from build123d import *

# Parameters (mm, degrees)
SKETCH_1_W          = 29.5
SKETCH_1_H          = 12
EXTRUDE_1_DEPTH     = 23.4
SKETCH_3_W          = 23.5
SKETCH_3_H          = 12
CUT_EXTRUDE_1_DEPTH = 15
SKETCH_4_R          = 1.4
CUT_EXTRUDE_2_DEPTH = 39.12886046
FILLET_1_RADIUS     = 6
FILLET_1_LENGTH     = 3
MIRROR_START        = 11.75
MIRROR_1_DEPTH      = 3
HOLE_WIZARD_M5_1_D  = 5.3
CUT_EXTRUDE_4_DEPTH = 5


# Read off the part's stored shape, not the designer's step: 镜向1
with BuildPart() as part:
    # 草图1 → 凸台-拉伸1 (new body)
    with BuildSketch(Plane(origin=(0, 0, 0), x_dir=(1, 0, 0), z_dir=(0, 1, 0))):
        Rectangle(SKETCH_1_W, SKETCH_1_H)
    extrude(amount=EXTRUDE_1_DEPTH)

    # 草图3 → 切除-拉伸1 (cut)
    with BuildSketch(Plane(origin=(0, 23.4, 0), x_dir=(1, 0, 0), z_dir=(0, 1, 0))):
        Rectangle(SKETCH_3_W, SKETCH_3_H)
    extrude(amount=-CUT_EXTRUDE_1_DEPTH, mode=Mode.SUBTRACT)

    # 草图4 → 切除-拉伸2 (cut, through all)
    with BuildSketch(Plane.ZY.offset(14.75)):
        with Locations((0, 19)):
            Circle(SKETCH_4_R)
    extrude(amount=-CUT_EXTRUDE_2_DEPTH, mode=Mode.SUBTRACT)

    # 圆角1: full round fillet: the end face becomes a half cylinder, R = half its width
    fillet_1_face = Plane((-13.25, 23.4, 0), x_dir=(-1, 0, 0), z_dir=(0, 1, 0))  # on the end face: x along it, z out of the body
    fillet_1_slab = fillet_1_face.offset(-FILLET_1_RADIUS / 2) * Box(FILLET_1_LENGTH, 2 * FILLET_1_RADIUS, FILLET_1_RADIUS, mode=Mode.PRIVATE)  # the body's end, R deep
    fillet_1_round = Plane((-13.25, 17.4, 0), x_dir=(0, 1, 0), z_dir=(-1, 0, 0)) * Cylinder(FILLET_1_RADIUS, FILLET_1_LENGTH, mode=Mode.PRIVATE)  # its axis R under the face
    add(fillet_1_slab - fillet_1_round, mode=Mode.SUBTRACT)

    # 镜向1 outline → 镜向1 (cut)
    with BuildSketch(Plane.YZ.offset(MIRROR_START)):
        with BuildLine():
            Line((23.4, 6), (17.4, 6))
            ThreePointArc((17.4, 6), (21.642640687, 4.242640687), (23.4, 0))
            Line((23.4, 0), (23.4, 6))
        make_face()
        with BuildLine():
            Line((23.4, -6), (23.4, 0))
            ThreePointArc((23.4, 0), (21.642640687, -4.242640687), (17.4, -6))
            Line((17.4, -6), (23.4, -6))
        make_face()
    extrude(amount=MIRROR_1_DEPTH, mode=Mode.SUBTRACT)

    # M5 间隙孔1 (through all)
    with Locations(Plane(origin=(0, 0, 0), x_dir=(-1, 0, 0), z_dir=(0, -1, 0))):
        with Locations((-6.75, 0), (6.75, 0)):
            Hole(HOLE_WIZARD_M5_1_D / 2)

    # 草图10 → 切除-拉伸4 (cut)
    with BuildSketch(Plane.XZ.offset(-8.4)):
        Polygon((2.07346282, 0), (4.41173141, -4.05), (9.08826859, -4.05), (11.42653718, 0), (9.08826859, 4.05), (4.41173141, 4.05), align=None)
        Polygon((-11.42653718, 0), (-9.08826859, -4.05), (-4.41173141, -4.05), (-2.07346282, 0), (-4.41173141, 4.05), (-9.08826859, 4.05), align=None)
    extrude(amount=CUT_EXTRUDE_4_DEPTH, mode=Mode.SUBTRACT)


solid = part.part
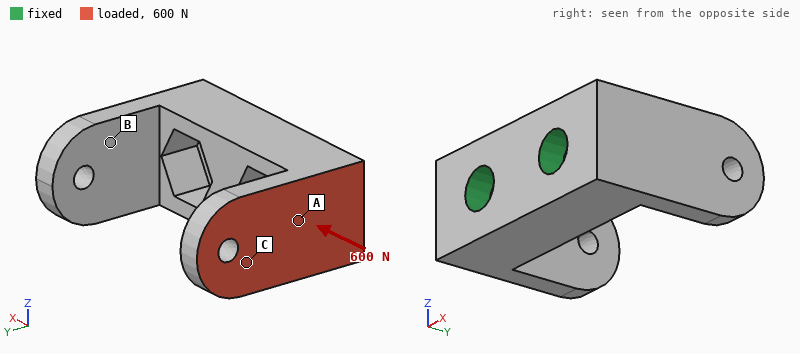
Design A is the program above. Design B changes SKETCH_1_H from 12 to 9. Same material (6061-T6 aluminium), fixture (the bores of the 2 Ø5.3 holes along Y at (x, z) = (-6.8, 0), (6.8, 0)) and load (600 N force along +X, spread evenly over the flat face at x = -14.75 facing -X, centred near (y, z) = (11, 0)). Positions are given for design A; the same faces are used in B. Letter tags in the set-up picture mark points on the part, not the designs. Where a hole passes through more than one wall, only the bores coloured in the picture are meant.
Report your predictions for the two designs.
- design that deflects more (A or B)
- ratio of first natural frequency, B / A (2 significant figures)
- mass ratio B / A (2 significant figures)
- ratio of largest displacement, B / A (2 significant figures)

B
0.88
0.70
1.6
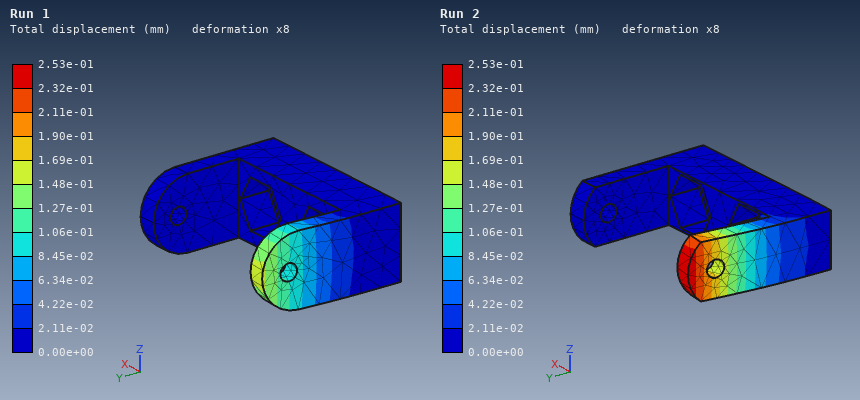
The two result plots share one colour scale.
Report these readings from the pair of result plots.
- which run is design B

Run 2
